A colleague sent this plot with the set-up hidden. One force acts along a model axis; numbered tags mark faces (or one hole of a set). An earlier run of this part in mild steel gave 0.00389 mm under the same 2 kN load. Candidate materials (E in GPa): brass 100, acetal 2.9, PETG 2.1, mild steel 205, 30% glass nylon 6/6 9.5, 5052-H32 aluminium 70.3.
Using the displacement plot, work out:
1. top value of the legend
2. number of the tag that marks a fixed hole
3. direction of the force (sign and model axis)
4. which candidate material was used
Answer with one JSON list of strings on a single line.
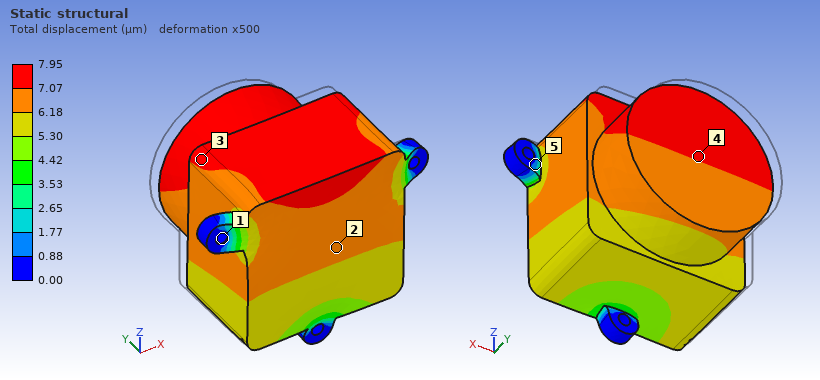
["7.95 µm", "1", "-Y", "brass"]
